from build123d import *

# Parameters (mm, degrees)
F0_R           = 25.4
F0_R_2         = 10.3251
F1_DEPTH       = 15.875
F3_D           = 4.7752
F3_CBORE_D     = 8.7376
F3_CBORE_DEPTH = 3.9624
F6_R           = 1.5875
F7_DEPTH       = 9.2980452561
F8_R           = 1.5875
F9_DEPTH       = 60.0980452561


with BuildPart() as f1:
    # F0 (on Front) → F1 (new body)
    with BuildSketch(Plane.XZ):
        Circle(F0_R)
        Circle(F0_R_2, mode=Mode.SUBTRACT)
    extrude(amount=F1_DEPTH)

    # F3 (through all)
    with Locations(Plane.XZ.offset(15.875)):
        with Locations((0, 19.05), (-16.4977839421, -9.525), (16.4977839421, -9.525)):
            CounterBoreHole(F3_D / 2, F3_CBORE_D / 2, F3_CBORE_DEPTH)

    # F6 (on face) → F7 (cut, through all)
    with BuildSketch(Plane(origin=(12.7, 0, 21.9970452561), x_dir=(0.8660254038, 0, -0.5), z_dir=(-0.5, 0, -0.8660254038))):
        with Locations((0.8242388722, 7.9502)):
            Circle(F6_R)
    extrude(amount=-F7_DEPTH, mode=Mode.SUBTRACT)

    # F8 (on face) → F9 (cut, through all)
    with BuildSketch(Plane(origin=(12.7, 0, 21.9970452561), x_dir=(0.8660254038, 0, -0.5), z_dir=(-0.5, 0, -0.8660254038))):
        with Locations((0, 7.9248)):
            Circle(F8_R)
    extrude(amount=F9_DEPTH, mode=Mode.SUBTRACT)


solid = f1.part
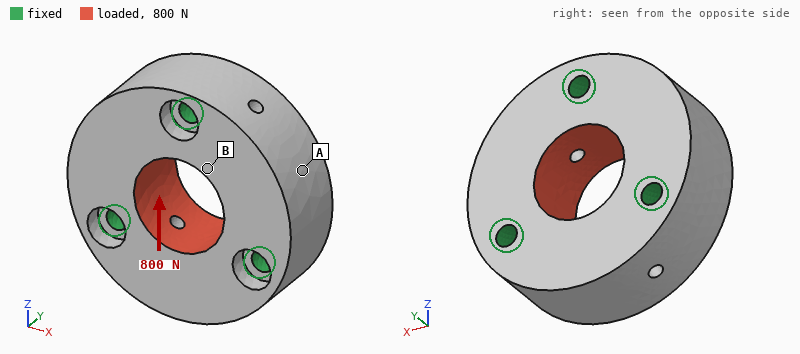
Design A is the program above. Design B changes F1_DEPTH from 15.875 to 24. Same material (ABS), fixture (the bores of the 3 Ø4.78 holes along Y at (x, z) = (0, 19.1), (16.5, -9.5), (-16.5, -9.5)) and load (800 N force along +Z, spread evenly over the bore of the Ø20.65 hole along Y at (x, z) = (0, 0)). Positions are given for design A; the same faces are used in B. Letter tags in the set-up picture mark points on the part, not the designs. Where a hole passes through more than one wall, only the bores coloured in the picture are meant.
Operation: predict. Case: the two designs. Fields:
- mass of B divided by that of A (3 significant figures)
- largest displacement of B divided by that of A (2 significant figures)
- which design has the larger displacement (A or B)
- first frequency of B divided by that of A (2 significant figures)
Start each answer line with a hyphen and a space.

- 1.49
- 1.4
- B
- 0.83
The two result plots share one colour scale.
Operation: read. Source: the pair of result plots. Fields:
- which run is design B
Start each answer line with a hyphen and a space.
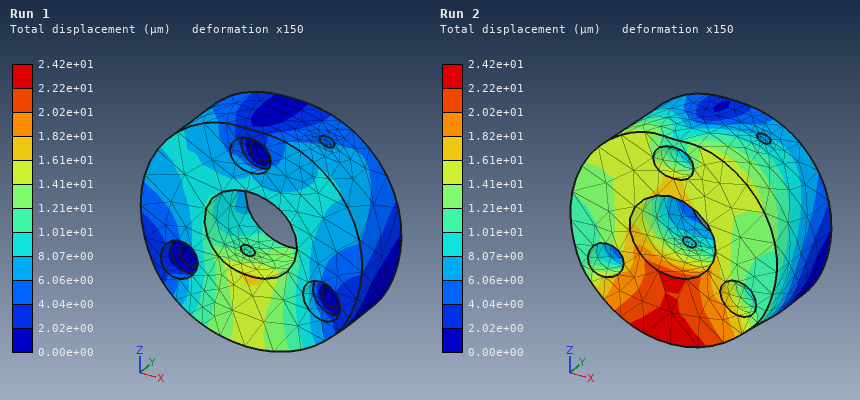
- Run 2
